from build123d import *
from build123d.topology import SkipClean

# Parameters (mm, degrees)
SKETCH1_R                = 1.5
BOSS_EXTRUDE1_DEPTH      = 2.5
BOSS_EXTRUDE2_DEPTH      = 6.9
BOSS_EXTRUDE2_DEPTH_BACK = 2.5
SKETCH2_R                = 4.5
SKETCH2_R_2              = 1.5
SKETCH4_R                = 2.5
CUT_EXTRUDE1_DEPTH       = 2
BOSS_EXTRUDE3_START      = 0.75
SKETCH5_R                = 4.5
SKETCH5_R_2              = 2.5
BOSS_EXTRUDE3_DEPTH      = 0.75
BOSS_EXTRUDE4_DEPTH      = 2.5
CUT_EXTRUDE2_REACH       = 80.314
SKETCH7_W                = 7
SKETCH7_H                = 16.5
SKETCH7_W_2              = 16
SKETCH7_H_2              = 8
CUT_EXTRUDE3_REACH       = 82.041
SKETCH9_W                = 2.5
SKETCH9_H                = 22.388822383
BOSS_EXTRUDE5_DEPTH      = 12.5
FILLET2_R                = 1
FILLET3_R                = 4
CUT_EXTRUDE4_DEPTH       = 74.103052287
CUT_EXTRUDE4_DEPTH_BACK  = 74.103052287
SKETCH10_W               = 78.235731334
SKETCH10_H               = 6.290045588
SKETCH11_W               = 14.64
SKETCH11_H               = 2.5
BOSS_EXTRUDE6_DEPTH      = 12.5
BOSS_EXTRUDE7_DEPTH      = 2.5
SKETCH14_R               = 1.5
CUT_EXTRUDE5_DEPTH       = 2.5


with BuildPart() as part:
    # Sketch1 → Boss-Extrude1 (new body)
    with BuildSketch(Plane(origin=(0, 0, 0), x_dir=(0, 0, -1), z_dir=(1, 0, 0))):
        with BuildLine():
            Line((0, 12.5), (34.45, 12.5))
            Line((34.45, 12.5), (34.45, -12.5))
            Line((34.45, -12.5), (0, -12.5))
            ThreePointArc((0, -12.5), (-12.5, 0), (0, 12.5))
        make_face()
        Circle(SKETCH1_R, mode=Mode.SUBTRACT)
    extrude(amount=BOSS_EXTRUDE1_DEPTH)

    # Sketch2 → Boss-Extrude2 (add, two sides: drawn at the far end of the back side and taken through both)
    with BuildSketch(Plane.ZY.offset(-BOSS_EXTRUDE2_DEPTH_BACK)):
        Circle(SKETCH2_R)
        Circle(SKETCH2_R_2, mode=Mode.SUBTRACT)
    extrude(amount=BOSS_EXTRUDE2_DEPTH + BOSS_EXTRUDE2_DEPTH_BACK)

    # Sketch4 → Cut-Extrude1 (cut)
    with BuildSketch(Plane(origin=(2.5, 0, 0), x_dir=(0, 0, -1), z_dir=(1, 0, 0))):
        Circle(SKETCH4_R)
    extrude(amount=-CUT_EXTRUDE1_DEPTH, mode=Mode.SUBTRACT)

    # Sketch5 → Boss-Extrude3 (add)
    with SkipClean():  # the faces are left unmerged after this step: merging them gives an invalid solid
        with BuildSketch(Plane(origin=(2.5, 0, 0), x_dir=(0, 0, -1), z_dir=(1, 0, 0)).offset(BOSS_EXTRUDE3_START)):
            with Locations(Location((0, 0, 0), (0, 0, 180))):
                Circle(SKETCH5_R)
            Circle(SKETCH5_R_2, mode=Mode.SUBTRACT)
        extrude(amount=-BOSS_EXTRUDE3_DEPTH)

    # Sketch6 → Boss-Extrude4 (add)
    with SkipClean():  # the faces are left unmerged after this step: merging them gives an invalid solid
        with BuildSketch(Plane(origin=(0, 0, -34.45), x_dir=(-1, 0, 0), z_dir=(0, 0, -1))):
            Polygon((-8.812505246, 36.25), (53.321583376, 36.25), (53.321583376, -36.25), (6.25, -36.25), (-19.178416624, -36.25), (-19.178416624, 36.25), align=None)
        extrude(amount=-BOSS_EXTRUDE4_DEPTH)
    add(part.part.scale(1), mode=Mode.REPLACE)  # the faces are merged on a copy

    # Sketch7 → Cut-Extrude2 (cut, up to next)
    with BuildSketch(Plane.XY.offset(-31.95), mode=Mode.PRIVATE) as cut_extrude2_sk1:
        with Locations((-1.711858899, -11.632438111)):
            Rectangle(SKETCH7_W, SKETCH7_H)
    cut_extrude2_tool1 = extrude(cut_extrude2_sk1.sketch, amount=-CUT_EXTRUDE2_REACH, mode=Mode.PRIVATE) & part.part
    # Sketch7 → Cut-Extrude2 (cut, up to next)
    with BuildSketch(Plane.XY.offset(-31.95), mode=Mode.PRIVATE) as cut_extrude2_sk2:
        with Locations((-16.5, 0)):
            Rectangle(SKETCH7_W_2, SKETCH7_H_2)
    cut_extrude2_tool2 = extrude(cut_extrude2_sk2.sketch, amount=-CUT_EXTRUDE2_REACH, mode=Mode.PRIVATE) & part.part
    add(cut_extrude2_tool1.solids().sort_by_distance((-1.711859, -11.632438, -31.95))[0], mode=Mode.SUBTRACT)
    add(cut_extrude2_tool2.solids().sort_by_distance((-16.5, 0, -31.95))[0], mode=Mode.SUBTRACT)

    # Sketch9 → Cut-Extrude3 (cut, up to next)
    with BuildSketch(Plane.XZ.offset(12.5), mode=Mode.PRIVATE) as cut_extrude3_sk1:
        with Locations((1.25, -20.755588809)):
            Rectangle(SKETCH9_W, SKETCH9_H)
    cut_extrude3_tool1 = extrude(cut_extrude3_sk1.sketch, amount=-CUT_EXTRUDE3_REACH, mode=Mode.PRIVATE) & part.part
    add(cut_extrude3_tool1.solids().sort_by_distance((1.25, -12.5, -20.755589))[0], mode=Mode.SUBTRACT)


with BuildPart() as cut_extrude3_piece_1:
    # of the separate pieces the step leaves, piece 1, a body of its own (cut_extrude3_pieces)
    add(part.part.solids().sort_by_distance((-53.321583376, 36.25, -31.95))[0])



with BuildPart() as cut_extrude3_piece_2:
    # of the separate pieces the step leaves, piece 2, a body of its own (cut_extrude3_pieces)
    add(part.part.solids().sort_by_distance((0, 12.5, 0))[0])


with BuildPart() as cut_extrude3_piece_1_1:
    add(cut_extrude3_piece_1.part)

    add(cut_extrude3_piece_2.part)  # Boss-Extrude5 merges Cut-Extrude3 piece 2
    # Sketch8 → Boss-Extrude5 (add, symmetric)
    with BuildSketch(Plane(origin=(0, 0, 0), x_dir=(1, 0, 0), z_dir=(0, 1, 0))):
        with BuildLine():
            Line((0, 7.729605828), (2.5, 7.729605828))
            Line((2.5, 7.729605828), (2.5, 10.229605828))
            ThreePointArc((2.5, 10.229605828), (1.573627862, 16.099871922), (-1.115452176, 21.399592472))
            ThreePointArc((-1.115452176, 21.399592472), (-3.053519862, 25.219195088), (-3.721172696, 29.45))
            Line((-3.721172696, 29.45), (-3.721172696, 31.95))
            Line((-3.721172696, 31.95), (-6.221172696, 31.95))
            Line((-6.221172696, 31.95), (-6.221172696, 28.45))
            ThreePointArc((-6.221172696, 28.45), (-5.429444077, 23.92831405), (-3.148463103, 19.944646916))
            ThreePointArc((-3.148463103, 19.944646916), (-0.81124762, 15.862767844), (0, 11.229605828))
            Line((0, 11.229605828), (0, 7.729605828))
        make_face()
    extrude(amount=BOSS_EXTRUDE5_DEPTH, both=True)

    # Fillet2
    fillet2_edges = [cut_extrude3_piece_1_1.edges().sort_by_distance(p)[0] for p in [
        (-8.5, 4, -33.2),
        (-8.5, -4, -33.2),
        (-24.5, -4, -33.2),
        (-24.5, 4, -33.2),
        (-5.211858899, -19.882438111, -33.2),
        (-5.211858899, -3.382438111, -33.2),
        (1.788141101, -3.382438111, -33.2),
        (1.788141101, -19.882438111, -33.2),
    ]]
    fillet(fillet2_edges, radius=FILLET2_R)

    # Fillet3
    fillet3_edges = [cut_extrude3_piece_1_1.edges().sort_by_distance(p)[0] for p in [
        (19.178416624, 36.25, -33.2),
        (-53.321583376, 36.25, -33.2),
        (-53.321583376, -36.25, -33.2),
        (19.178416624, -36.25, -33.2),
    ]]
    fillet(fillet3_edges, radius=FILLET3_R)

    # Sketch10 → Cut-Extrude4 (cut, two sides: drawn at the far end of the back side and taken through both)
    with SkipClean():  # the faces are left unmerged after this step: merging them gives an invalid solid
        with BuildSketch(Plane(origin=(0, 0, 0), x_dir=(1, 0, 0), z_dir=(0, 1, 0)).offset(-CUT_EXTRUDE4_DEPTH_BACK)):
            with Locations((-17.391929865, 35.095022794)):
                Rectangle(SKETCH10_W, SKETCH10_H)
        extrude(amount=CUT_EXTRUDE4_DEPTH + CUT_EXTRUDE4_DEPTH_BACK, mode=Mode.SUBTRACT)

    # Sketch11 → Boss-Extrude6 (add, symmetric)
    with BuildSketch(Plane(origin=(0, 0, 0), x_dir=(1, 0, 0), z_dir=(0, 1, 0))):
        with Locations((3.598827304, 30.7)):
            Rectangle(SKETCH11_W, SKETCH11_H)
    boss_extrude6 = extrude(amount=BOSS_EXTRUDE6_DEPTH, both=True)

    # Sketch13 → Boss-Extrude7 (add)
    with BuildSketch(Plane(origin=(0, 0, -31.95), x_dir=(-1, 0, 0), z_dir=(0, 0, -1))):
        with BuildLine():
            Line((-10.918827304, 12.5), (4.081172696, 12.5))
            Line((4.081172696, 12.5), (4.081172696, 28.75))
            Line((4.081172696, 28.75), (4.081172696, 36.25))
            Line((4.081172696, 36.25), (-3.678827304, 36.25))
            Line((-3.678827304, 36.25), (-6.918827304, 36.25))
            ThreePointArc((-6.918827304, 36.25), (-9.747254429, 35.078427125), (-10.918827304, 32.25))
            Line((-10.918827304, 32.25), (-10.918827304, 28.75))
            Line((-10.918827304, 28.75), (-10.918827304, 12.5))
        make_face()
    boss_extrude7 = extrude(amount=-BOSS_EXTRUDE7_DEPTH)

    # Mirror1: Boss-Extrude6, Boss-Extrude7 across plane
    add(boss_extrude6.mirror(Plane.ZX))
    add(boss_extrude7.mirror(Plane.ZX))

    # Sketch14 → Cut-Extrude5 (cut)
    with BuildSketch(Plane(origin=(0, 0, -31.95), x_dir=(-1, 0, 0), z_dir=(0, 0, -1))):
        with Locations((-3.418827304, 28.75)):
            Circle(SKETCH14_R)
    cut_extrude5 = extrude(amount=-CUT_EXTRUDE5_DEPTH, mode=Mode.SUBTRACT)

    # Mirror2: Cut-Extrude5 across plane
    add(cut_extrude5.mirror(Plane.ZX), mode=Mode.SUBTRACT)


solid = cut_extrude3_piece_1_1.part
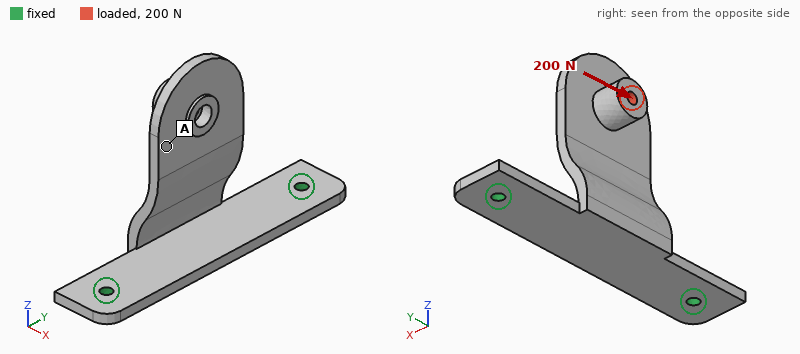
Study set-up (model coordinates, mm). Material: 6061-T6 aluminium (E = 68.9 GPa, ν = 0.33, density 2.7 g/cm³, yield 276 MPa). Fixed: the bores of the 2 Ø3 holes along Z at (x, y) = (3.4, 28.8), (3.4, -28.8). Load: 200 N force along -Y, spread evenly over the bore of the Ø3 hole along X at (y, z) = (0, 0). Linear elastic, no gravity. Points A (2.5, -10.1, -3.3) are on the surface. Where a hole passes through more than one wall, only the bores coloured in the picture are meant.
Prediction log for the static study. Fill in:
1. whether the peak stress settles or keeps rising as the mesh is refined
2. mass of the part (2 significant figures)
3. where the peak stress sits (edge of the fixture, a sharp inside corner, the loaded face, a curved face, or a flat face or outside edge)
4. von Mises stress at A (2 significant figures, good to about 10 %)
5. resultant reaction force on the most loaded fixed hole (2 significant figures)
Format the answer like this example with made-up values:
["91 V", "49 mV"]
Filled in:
["keeps rising", "15 g", "a sharp inside corner", "21 MPa", "180 N"]
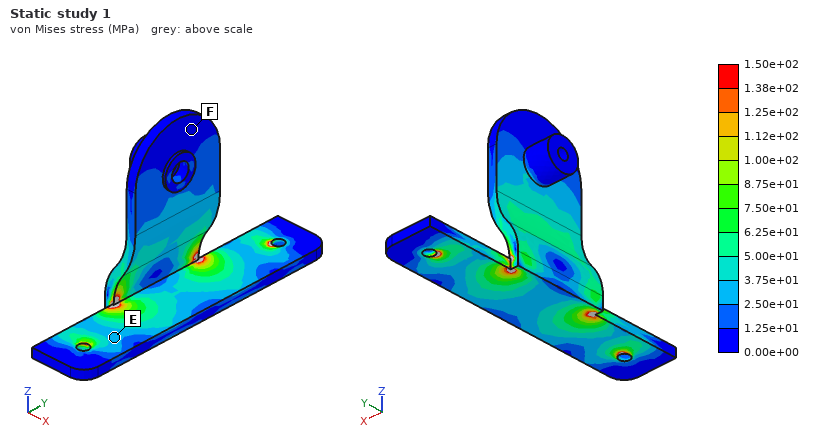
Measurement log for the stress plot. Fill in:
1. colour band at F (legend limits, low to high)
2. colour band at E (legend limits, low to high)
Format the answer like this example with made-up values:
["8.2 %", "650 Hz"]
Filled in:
["0.00e+00 to 1.25e+01 MPa", "2.50e+01 to 3.75e+01 MPa"]
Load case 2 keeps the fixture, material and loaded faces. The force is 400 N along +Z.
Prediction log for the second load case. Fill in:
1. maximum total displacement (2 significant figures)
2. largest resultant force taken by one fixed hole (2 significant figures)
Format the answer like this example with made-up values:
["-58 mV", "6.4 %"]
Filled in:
["0.79 mm", "210 N"]
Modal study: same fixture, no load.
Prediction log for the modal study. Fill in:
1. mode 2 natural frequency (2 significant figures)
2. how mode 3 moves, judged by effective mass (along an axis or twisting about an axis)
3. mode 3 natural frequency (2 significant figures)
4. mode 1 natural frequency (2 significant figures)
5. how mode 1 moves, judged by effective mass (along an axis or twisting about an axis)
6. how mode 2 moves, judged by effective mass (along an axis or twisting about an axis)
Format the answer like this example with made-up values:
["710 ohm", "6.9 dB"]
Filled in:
["1900 Hz", "along Z", "2400 Hz", "700 Hz", "along X", "along Y"]
